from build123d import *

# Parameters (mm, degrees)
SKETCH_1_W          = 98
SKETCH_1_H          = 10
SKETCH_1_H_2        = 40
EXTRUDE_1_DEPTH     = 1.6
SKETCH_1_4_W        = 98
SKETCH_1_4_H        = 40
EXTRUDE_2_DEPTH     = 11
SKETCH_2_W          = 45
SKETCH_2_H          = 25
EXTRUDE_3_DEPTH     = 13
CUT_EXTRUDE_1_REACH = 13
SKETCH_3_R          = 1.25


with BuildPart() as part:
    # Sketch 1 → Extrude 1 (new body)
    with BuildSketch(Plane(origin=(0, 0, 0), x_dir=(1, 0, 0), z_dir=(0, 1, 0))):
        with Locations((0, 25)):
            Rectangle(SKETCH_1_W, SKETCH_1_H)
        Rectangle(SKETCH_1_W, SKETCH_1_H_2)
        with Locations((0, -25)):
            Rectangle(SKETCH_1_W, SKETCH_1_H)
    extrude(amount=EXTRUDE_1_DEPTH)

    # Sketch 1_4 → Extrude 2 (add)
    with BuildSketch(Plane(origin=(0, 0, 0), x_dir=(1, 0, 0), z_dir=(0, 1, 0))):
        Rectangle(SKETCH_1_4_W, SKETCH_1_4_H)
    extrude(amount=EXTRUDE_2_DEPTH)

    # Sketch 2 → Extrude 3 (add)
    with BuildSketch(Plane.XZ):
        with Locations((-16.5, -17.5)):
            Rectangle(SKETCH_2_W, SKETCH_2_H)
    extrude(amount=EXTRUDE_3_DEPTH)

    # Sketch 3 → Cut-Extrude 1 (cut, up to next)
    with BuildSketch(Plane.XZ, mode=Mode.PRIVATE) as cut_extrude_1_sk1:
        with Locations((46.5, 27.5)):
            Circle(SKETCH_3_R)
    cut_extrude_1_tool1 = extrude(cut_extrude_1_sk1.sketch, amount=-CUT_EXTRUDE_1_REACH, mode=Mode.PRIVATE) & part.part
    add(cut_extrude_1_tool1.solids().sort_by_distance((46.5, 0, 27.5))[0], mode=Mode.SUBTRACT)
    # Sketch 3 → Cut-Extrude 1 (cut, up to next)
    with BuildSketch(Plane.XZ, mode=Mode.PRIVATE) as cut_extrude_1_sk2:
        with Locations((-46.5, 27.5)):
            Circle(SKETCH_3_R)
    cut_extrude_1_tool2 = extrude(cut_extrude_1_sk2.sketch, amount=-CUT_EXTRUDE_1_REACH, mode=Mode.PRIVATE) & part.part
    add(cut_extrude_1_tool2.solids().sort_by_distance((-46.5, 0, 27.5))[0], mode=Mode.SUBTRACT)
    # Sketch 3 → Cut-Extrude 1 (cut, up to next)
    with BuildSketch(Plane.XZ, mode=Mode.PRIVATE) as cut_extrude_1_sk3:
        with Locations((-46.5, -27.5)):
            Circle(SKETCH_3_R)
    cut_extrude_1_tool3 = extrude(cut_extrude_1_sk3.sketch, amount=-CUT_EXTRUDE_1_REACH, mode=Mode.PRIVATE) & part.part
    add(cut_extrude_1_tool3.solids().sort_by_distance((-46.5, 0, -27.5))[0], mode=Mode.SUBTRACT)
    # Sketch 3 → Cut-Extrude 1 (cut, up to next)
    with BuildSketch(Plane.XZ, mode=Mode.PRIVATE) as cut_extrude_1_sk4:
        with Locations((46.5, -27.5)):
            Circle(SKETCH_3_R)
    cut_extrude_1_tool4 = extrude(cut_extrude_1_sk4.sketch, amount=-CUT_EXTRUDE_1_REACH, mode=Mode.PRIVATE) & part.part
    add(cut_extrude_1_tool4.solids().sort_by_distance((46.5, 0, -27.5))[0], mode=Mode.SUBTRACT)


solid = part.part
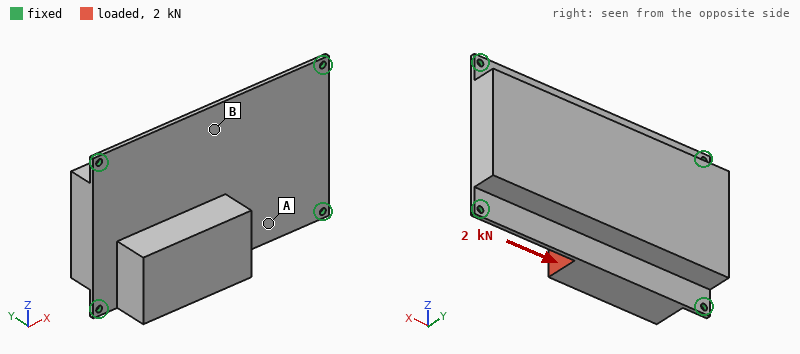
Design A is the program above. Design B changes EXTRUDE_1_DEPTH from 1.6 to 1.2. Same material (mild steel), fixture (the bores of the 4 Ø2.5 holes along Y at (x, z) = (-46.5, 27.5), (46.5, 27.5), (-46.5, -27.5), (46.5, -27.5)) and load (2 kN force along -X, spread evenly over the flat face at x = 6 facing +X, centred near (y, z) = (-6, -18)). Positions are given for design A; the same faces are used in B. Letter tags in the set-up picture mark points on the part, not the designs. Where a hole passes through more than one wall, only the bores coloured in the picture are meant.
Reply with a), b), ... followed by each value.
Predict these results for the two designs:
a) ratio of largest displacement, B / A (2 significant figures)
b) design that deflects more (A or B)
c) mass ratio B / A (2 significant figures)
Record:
a) 1.3
b) B
c) 0.99
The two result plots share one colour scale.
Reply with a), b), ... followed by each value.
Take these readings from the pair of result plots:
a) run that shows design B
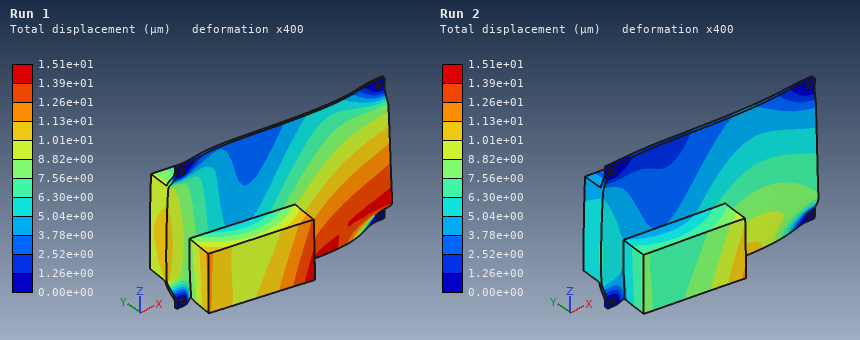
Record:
a) Run 1
